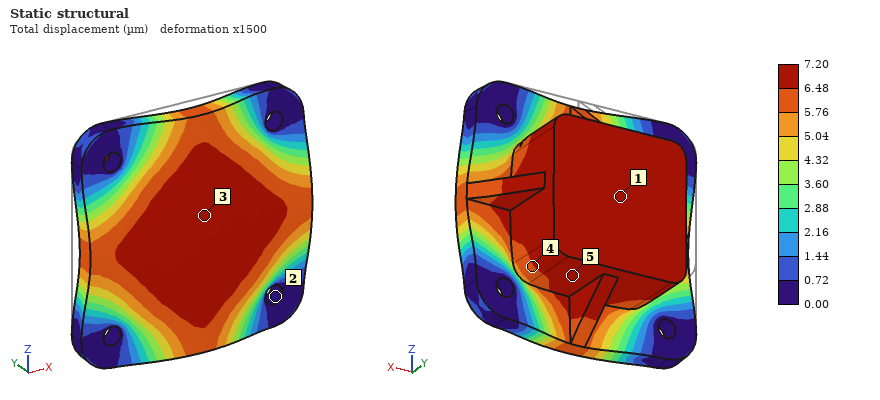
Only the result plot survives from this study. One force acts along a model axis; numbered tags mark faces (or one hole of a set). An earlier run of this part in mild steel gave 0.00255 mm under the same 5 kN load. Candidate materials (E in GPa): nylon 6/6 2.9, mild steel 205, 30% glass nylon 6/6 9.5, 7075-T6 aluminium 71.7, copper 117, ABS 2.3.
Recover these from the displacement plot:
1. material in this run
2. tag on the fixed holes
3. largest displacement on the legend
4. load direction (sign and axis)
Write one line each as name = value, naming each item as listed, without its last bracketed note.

material in this run = 7075-T6 aluminium
tag on the fixed holes = 2
largest displacement on the legend = 7.20 µm
load direction = -Y
